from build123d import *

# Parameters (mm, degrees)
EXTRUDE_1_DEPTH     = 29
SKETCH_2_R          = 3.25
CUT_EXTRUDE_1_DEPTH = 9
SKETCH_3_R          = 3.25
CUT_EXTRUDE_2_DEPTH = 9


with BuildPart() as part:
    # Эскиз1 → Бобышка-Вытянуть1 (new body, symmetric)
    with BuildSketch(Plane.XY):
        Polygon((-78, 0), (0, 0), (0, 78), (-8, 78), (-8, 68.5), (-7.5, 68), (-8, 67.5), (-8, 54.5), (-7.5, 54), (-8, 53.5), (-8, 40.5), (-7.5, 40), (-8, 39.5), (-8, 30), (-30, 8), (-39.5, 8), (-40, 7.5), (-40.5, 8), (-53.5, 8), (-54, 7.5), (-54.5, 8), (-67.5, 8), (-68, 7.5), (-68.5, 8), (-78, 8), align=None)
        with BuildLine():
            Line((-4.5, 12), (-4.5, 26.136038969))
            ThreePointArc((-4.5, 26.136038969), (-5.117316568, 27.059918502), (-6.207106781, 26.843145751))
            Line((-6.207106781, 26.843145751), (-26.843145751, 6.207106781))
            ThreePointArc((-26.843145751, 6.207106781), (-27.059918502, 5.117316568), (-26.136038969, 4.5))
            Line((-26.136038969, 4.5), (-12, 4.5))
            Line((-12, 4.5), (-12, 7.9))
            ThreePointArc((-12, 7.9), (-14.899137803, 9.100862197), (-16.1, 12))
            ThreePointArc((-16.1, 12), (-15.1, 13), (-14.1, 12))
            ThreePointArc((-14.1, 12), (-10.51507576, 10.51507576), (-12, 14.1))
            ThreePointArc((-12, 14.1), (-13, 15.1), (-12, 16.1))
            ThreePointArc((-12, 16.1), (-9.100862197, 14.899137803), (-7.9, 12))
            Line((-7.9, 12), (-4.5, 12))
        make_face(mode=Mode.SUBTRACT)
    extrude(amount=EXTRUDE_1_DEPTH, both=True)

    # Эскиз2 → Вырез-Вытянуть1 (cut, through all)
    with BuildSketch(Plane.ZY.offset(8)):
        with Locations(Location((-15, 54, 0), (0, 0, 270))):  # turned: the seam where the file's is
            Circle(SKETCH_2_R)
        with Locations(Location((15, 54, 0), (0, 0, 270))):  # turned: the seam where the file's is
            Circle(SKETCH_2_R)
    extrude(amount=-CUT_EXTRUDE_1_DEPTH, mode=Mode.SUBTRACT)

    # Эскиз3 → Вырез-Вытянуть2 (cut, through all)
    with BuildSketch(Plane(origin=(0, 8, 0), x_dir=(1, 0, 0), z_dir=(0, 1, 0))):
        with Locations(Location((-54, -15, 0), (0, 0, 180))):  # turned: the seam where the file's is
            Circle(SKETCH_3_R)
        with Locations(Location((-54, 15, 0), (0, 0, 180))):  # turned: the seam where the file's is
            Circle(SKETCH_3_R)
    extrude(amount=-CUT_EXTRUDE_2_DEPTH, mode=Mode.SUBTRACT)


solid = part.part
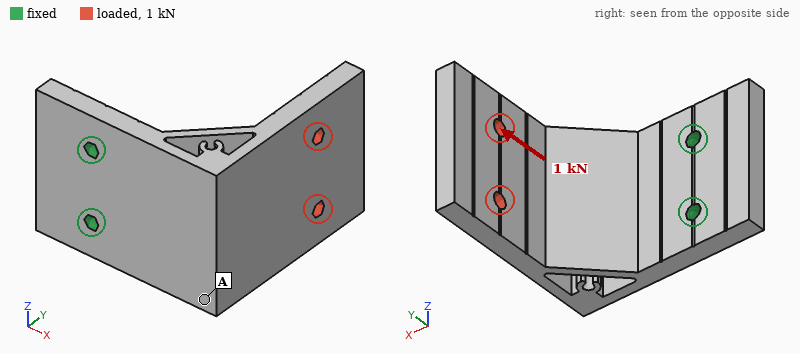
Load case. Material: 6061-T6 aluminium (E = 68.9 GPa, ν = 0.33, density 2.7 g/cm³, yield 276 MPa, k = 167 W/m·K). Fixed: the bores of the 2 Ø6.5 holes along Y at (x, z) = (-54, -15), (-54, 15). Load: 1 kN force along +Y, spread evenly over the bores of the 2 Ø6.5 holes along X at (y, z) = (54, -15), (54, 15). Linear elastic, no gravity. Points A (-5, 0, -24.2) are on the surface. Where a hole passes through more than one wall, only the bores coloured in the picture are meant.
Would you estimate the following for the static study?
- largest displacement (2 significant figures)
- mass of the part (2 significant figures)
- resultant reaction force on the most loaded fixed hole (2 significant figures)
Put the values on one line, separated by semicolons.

0.65 mm; 190 g; 500 N
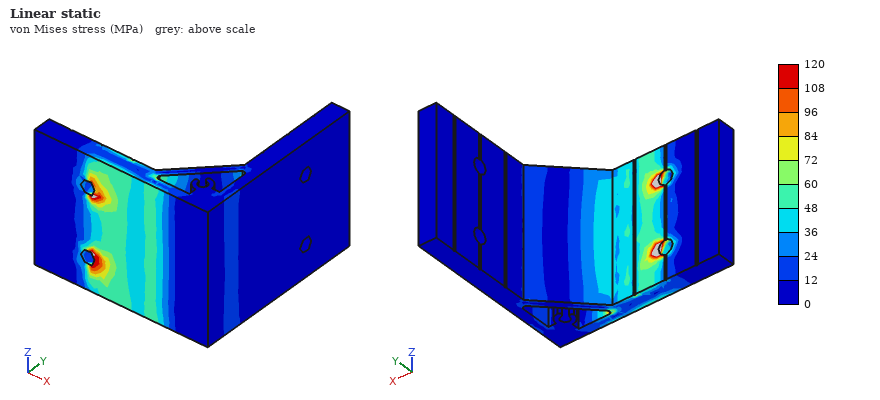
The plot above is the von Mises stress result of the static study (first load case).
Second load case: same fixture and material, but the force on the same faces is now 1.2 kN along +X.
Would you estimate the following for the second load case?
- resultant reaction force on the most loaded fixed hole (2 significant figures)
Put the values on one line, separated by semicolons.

620 N
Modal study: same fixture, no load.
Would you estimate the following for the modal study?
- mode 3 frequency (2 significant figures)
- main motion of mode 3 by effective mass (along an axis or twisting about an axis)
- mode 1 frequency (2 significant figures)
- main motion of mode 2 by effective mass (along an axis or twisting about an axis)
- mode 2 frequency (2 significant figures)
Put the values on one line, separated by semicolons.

2300 Hz; along Y; 600 Hz; along Z; 1500 Hz
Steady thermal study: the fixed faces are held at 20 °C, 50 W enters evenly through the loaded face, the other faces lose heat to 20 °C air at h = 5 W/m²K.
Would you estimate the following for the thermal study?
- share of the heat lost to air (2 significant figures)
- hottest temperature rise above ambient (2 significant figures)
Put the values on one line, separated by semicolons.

6.9 %; 58 K
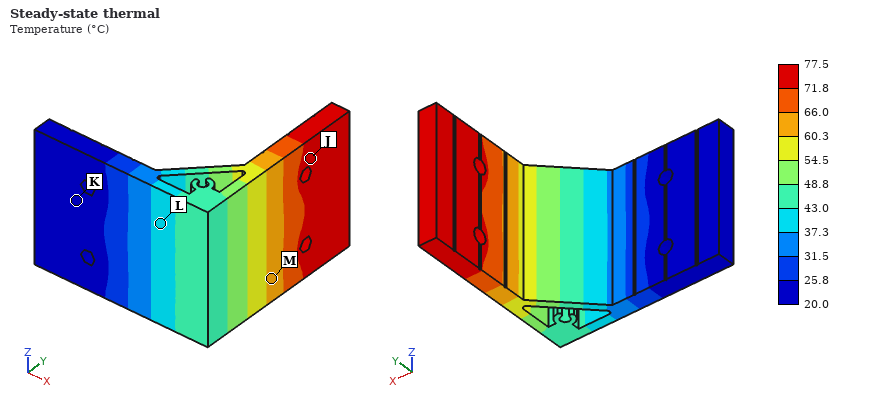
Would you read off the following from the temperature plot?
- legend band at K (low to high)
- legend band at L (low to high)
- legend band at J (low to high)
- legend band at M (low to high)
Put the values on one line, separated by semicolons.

20.0 to 25.8 °C; 37.3 to 43.0 °C; 71.8 to 77.5 °C; 60.3 to 66.0 °C
